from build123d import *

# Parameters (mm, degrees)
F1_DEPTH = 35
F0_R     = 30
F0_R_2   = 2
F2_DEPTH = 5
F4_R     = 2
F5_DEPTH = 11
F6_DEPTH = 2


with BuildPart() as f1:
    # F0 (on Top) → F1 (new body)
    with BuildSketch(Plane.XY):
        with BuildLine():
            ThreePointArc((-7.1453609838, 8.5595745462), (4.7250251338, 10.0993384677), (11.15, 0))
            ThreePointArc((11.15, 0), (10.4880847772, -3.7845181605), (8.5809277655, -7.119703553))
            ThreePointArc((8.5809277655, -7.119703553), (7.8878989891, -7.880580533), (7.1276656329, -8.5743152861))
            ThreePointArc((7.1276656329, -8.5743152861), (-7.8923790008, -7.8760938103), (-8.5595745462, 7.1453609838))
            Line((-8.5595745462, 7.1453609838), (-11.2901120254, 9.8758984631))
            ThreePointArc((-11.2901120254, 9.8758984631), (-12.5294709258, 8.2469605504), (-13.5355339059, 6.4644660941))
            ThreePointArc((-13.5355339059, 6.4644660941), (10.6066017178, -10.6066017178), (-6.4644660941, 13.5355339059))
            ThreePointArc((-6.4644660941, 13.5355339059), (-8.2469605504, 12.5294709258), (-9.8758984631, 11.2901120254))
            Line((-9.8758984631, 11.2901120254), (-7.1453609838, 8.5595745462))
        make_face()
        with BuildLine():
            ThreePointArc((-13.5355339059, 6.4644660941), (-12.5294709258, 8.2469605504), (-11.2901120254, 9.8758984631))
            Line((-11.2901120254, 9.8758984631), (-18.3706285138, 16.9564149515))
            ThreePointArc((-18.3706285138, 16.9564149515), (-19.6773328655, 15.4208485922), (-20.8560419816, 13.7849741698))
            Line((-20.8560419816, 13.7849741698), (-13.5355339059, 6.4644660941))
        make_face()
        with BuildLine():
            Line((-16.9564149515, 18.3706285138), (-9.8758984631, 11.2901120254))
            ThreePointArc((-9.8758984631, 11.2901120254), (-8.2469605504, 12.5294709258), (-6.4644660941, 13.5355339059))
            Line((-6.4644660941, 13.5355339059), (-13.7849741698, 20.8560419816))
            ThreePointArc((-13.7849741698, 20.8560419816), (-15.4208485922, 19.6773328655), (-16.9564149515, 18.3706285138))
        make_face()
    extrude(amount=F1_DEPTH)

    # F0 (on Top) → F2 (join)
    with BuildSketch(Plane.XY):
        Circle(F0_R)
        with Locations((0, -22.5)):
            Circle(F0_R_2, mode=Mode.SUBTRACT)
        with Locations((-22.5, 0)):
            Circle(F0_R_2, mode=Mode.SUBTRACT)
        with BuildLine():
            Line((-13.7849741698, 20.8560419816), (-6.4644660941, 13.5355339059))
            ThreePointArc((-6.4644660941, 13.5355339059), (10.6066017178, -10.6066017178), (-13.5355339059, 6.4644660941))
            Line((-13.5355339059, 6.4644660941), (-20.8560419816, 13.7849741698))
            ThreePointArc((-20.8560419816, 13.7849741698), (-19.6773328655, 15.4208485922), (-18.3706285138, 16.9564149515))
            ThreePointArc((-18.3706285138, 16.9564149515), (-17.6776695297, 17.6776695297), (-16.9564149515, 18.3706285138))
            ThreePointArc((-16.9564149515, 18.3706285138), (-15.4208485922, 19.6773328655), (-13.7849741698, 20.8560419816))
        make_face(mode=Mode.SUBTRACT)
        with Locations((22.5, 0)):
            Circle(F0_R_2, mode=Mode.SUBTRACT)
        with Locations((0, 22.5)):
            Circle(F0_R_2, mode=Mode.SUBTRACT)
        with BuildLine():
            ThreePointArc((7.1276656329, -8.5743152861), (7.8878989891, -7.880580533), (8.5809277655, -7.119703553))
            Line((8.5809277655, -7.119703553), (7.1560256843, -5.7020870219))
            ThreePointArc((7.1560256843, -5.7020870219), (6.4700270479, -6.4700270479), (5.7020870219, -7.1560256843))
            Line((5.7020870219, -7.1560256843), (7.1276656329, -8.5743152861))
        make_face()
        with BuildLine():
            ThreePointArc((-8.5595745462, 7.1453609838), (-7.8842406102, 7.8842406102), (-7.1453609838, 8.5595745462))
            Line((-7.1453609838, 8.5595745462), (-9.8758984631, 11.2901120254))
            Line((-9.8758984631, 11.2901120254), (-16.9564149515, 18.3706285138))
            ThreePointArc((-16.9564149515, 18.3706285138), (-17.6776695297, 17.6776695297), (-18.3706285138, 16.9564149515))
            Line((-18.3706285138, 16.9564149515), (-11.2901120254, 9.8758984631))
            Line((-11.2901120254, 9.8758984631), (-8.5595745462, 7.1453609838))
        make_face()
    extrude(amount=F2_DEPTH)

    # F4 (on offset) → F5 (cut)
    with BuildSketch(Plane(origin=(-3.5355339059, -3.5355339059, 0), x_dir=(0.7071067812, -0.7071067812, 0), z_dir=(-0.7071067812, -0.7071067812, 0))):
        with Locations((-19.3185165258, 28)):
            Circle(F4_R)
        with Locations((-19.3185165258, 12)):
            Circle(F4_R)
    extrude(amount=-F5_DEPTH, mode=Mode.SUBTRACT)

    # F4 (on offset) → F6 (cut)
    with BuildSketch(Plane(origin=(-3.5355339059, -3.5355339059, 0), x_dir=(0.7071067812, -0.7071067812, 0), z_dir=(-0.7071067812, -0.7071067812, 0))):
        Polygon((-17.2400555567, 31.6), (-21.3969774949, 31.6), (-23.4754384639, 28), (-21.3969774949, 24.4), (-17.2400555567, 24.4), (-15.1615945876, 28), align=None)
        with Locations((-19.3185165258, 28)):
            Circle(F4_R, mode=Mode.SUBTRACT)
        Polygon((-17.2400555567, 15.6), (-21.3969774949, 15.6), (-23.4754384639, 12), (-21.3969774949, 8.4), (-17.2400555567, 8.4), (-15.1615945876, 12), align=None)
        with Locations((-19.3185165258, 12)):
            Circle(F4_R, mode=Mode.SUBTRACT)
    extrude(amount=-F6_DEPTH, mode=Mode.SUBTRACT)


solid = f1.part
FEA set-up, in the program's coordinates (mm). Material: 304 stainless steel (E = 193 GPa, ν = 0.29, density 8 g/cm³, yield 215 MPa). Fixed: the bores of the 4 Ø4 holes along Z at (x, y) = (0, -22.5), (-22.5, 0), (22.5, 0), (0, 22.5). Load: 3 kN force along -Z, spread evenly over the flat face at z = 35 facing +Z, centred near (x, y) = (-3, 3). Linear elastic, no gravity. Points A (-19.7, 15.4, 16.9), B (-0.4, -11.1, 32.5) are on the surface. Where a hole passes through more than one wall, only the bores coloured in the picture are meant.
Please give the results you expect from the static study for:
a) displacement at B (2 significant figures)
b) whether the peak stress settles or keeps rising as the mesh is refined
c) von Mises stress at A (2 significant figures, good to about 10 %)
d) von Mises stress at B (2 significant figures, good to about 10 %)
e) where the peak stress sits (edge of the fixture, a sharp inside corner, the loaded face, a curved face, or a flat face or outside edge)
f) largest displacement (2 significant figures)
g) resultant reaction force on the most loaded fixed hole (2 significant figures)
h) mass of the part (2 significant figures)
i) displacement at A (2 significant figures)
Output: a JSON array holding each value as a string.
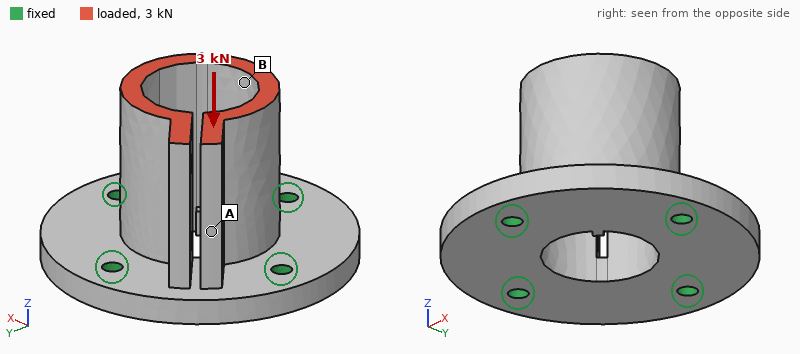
["4.0 µm", "keeps rising", "16 MPa", "7.8 MPa", "edge of the fixture", "9.8 µm", "940 N", "190 g", "6.5 µm"]
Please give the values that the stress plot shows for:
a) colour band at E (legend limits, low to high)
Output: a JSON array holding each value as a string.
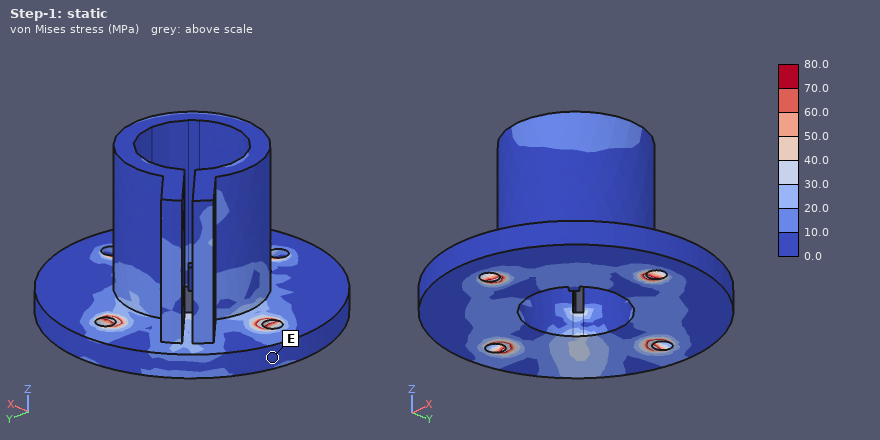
["0.0 to 10.0 MPa"]
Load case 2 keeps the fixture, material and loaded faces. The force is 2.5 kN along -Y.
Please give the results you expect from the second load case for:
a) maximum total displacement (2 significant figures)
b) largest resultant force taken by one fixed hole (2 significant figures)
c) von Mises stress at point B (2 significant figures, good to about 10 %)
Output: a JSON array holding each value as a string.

["97 µm", "2.2 kN", "28 MPa"]
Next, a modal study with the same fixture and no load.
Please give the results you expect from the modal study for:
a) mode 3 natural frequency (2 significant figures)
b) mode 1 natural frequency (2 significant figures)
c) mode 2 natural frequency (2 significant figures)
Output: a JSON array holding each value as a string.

["8100 Hz", "5000 Hz", "6100 Hz"]
